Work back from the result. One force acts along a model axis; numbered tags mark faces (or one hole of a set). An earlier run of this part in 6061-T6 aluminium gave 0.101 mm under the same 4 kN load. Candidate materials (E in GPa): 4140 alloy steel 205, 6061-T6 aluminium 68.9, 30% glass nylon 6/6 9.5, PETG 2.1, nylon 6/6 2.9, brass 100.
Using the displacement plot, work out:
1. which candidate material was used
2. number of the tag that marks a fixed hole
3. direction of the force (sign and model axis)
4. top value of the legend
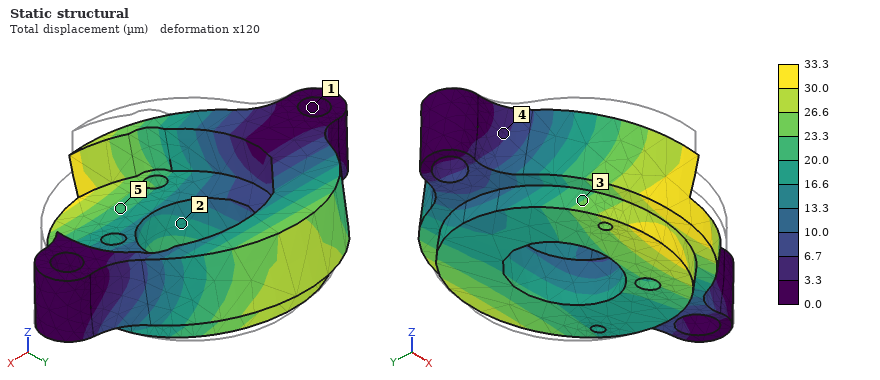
4140 alloy steel
1
+Y
33.3 µm
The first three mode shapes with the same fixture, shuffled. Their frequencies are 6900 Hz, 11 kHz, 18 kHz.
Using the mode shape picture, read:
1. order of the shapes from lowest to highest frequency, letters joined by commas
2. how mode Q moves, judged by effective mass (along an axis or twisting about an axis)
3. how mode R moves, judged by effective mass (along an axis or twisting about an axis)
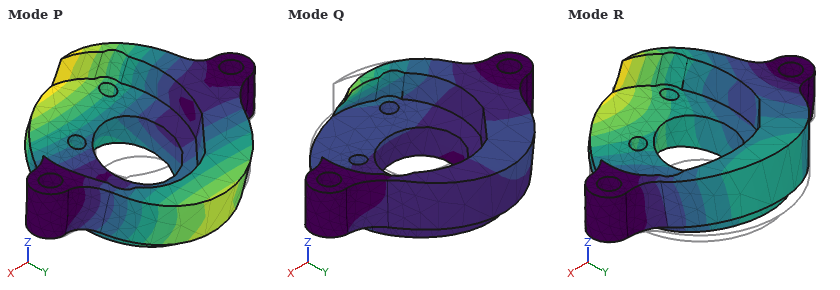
P, R, Q
along Y
along Z
